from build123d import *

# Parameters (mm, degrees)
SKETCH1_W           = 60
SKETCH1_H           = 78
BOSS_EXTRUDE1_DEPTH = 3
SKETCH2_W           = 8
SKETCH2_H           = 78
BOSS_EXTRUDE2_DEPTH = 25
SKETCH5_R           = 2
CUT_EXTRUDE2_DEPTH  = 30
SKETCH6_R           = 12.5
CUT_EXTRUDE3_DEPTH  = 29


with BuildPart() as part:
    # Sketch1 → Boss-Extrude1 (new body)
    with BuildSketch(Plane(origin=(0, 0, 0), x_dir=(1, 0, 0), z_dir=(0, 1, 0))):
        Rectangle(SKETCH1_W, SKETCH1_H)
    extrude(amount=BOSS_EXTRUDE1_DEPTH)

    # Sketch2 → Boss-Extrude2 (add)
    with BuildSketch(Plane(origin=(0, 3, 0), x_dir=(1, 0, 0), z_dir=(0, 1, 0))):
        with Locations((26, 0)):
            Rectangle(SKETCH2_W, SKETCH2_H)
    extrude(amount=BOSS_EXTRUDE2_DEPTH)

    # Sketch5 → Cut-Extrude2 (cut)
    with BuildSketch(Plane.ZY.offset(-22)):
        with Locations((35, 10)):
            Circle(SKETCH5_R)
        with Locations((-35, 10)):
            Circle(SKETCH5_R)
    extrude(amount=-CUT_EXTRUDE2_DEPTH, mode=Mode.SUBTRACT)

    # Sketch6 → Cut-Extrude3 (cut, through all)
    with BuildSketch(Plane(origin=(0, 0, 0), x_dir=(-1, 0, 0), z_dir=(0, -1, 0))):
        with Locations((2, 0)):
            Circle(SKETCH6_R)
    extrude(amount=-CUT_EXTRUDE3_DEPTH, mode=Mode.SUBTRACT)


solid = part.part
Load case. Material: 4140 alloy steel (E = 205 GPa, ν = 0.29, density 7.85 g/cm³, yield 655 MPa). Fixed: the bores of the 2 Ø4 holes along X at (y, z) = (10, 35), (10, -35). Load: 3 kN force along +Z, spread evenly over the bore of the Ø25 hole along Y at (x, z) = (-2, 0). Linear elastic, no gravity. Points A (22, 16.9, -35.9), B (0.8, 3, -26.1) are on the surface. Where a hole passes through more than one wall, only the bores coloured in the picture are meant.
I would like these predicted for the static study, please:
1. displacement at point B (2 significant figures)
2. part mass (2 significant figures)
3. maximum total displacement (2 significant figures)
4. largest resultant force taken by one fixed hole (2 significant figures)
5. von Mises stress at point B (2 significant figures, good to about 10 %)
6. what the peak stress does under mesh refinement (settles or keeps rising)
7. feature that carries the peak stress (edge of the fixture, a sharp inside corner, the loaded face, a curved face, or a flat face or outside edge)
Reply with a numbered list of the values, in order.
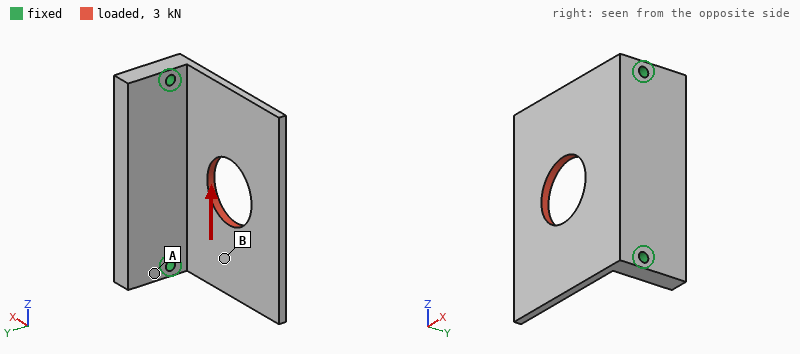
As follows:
1. 11 µm
2. 220 g
3. 22 µm
4. 2.0 kN
5. 24 MPa
6. keeps rising
7. edge of the fixture
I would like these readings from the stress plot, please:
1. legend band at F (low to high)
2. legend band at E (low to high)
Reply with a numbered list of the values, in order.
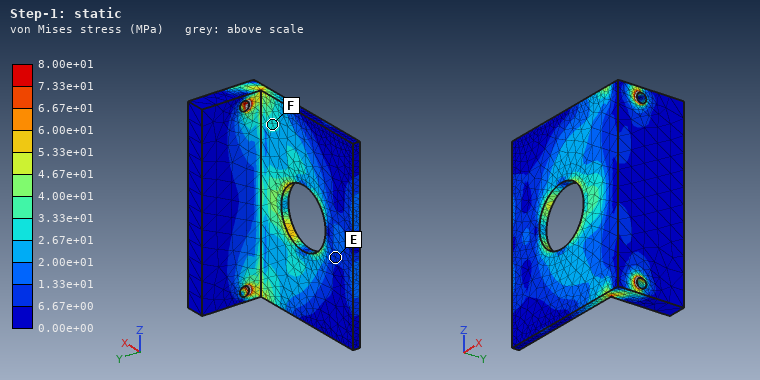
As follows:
1. 2.67e+01 to 3.33e+01 MPa
2. 6.67e+00 to 1.33e+01 MPa
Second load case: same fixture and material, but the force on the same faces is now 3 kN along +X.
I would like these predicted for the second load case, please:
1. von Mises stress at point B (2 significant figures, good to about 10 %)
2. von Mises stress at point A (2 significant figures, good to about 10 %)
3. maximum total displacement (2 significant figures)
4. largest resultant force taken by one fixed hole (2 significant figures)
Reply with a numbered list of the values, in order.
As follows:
1. 18 MPa
2. 15 MPa
3. 32 µm
4. 1.6 kN
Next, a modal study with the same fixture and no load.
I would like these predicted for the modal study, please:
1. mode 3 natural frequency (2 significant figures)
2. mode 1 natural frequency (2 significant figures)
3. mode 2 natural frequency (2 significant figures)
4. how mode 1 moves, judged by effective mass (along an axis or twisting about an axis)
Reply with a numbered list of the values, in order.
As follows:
1. 3600 Hz
2. 810 Hz
3. 1500 Hz
4. along Y
